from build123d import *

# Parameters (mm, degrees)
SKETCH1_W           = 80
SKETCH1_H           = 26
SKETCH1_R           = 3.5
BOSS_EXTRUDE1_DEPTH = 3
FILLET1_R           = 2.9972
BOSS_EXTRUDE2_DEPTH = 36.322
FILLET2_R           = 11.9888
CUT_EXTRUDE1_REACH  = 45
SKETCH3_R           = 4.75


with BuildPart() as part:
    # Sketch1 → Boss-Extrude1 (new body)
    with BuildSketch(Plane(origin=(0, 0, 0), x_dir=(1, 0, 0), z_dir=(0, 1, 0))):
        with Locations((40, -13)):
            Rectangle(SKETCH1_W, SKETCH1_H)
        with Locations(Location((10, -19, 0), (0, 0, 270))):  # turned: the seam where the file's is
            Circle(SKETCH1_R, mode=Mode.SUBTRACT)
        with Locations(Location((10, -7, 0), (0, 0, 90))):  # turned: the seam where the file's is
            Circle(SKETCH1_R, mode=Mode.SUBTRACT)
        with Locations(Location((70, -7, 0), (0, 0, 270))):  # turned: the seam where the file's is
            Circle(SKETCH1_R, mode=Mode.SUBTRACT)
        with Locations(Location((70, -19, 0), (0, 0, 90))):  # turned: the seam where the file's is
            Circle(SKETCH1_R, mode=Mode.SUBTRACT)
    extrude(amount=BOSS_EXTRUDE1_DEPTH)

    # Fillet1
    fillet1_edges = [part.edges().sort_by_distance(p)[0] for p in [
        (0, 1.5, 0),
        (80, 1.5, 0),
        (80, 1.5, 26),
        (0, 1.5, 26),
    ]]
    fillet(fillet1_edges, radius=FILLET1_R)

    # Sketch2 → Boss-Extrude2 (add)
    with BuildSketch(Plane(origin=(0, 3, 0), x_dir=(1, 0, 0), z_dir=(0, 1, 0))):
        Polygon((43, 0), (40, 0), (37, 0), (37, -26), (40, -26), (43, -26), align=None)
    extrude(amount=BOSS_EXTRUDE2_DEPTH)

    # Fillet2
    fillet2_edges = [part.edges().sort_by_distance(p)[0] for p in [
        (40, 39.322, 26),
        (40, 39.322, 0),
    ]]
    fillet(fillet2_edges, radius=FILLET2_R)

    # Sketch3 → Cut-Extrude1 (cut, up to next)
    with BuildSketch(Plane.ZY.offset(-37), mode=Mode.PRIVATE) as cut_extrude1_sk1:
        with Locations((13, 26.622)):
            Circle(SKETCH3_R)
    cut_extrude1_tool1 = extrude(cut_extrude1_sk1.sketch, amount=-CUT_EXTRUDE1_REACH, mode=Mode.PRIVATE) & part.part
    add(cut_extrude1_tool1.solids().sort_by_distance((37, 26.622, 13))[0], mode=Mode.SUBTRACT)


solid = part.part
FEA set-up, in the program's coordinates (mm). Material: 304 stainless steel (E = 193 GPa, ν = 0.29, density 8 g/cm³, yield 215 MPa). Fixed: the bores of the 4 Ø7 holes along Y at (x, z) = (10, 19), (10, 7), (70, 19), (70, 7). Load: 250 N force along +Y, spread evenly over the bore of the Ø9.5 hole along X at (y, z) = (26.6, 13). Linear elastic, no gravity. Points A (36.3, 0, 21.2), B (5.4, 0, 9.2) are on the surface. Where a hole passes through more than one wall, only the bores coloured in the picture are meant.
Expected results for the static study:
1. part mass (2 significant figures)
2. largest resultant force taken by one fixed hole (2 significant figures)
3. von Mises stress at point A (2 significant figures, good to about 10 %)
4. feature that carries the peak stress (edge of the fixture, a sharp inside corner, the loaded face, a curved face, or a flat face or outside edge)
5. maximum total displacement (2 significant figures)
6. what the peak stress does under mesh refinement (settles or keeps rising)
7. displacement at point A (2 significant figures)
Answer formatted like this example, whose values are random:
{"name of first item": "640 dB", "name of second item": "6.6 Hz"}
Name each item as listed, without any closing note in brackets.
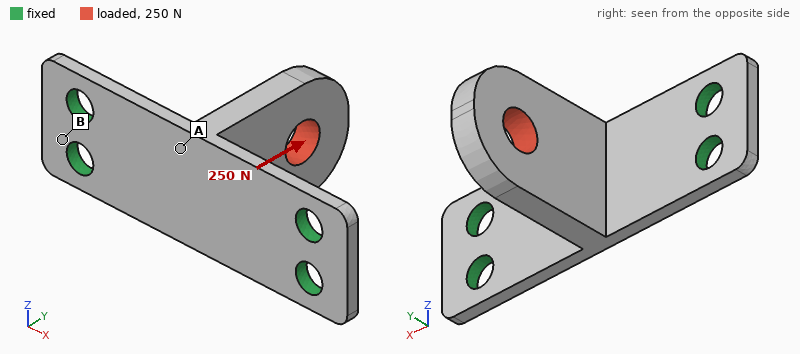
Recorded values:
{"part mass": "85 g", "largest resultant force taken by one fixed hole": "66 N", "von Mises stress at point A": "29 MPa", "feature that carries the peak stress": "edge of the fixture", "maximum total displacement": "16 µm", "what the peak stress does under mesh refinement": "keeps rising", "displacement at point A": "15 µm"}
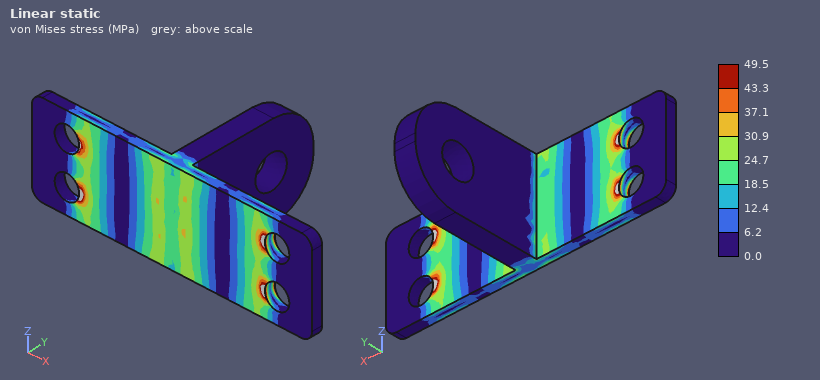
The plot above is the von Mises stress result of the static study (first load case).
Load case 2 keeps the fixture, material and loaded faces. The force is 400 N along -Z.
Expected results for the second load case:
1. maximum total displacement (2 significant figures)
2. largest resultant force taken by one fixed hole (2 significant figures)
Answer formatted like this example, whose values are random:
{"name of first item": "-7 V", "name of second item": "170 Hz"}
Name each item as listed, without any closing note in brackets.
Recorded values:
{"maximum total displacement": "0.18 mm", "largest resultant force taken by one fixed hole": "360 N"}
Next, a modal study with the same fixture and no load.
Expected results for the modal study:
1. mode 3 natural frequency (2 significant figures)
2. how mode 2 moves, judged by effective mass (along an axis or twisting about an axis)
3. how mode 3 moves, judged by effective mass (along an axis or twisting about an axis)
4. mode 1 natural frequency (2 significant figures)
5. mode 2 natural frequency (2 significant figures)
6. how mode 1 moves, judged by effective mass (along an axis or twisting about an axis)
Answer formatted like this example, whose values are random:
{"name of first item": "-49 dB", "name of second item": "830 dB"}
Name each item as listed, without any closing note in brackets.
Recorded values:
{"mode 3 natural frequency": "2800 Hz", "how mode 2 moves, judged by effective mass": "along X", "how mode 3 moves, judged by effective mass": "along Y", "mode 1 natural frequency": "1700 Hz", "mode 2 natural frequency": "2200 Hz", "how mode 1 moves, judged by effective mass": "along Z"}
